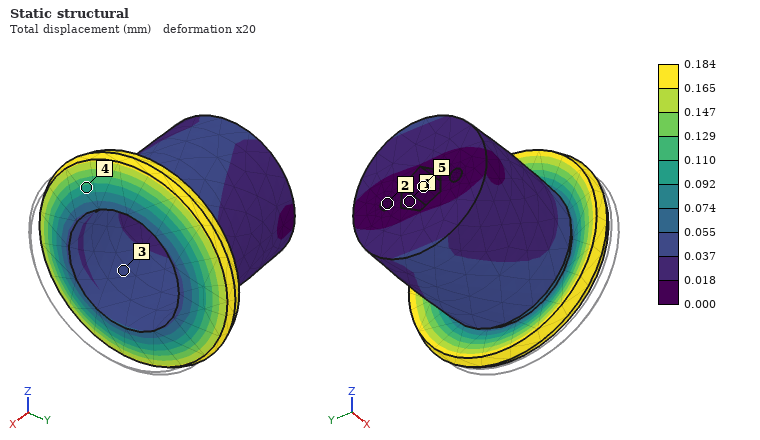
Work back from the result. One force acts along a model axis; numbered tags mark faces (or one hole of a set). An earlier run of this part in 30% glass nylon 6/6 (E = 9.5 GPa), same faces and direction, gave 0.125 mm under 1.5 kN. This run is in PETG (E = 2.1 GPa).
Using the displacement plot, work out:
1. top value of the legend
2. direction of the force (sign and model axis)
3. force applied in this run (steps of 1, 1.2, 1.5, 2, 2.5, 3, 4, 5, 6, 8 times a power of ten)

0.184 mm
-X
500 N
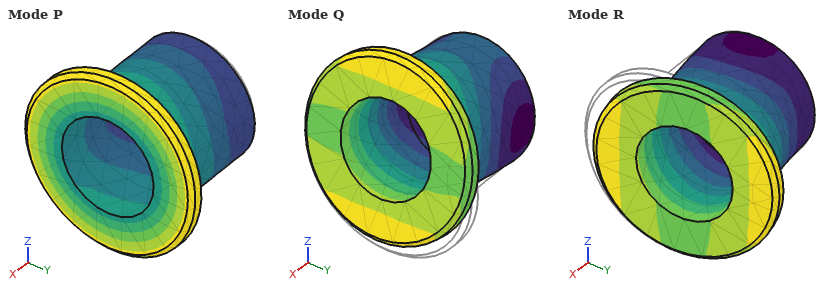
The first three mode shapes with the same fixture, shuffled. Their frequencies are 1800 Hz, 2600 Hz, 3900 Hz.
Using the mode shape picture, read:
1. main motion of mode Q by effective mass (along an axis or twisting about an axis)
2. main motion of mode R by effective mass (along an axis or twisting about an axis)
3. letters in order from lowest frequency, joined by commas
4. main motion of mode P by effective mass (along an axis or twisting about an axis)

along Z
along Y
Q, R, P
twisting about X
